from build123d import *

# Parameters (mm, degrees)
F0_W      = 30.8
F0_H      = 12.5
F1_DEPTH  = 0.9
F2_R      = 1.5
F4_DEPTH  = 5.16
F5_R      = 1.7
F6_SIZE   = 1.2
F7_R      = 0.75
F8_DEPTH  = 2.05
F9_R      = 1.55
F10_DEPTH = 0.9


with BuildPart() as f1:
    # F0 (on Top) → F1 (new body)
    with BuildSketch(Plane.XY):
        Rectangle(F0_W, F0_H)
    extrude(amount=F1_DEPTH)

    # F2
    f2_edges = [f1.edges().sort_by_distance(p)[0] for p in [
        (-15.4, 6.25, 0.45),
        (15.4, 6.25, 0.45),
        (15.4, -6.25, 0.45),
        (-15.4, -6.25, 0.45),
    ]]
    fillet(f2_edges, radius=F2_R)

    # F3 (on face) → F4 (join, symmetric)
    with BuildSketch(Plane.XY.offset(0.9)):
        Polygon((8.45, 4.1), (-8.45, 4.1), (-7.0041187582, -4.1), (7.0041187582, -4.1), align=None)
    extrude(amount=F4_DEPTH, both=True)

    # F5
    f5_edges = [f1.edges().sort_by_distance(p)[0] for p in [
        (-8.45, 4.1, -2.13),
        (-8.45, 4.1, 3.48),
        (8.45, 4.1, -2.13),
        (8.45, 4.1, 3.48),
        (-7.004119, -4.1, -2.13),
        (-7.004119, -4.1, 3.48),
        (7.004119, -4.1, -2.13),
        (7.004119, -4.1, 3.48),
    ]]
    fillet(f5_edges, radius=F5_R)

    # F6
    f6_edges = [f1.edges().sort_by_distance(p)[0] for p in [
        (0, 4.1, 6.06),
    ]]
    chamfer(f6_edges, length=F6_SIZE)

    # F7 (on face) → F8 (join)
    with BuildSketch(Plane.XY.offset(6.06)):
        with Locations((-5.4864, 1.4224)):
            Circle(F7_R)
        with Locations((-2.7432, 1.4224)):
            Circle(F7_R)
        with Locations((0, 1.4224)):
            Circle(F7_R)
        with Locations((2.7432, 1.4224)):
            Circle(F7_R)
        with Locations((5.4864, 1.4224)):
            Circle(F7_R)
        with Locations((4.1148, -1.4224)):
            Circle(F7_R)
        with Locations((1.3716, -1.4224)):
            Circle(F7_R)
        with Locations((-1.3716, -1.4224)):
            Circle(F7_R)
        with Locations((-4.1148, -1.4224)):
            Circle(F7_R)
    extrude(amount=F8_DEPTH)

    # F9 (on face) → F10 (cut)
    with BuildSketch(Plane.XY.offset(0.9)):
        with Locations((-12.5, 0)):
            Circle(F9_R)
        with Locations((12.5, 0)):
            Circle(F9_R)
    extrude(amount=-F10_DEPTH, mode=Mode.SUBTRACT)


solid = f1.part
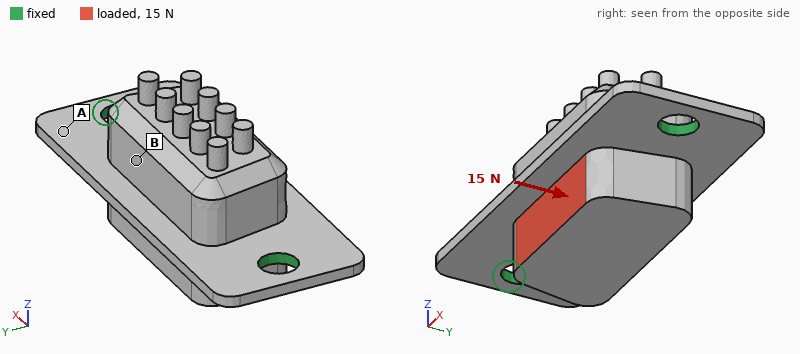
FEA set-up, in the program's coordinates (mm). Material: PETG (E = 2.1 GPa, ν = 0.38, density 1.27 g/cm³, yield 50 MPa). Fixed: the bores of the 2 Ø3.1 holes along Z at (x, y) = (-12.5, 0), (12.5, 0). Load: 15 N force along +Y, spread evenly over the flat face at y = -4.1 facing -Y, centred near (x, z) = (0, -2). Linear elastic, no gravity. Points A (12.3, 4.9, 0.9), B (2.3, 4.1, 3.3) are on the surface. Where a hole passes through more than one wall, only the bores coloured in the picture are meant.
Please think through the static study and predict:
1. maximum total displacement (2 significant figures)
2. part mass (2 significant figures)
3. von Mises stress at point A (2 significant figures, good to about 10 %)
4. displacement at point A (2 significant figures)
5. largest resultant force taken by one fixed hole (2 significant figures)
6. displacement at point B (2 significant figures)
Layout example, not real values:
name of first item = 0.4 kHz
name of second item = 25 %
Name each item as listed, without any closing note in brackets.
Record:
maximum total displacement = 0.15 mm
part mass = 1.9 g
von Mises stress at point A = 3.1 MPa
displacement at point A = 0.032 mm
largest resultant force taken by one fixed hole = 7.5 N
displacement at point B = 0.086 mm
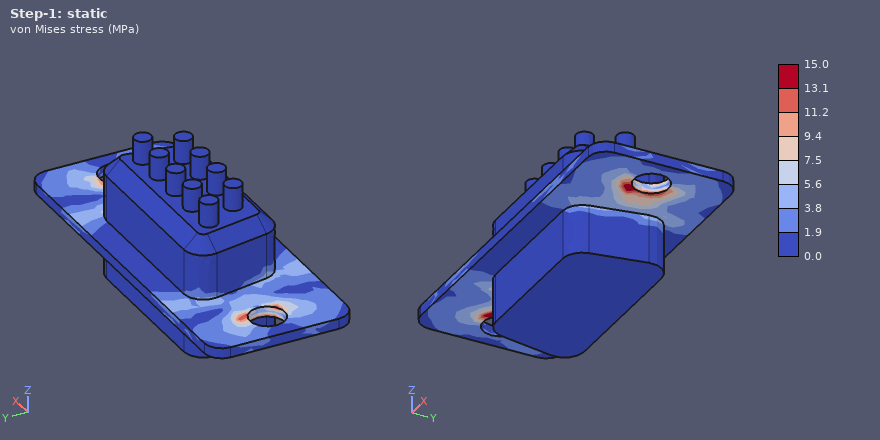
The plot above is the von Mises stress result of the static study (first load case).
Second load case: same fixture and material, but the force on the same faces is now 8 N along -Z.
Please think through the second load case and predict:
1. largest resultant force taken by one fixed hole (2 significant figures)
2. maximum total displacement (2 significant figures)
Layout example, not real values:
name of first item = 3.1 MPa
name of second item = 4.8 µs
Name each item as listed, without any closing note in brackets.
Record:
largest resultant force taken by one fixed hole = 4.0 N
maximum total displacement = 0.15 mm
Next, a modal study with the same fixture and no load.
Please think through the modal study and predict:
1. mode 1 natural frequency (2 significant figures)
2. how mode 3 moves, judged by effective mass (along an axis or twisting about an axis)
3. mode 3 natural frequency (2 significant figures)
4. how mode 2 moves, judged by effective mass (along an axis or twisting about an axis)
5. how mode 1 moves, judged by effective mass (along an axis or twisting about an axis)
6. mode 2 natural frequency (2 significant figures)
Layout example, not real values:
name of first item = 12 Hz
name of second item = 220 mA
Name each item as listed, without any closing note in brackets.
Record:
mode 1 natural frequency = 1400 Hz
how mode 3 moves, judged by effective mass = twisting about Y
mode 3 natural frequency = 4100 Hz
how mode 2 moves, judged by effective mass = along Z
how mode 1 moves, judged by effective mass = twisting about X
mode 2 natural frequency = 2300 Hz
